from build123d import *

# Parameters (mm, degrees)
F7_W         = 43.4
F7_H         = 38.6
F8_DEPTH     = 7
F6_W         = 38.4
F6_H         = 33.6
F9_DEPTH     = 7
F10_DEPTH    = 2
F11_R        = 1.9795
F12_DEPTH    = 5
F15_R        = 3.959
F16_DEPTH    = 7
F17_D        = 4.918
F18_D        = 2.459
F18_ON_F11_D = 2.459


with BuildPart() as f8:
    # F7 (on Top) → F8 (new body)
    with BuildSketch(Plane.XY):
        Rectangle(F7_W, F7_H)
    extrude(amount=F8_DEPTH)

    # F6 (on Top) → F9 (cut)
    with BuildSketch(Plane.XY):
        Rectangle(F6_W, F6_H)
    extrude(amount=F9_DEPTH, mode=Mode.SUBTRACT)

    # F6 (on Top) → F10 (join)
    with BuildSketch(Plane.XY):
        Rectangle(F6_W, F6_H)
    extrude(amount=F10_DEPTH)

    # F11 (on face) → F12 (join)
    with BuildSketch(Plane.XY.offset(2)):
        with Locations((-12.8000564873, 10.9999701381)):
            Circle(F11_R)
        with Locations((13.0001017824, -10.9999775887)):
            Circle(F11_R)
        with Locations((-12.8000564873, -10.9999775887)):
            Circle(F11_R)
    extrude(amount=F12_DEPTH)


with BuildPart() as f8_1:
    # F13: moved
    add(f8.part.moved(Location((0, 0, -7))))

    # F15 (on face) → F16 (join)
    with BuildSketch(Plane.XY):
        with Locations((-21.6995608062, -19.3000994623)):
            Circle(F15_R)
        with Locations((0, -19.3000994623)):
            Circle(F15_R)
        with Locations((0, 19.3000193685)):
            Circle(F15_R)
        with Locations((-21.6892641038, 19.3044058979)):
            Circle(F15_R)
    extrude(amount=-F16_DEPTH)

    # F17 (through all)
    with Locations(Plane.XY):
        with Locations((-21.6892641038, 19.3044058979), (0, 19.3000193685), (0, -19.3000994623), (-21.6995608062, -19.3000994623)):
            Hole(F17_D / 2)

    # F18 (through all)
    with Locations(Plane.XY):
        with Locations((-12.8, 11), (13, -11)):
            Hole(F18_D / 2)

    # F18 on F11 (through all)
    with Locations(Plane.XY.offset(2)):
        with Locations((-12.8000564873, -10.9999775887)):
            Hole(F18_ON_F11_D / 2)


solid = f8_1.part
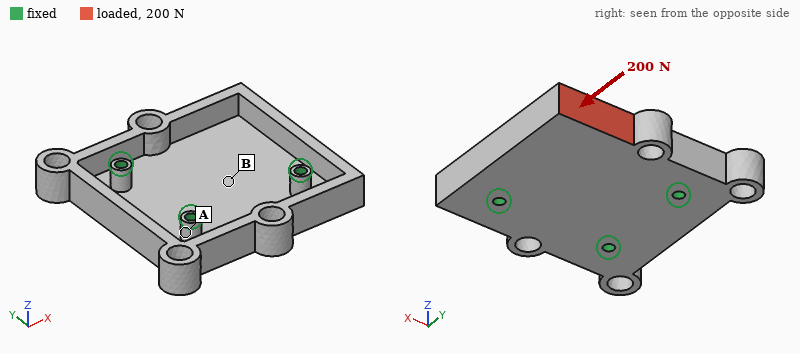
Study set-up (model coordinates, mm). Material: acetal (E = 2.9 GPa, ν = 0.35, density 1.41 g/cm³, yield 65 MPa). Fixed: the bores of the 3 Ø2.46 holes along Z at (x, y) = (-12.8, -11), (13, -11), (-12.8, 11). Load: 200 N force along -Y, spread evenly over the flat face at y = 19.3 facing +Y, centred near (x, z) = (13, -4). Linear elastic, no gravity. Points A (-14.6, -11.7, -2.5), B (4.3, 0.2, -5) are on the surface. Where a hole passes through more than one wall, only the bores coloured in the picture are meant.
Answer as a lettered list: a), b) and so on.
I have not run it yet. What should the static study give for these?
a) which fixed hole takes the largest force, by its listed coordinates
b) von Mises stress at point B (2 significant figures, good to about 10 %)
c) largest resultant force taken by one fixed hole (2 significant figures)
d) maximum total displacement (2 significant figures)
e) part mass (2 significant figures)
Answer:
a) (13, -11)
b) 5.3 MPa
c) 170 N
d) 0.68 mm
e) 8.1 g
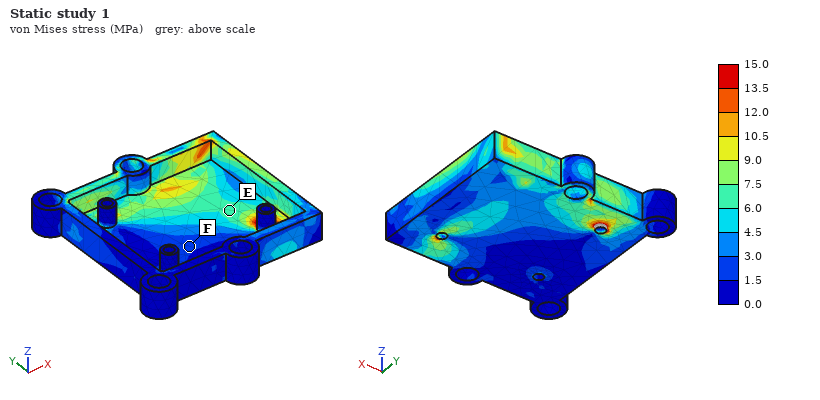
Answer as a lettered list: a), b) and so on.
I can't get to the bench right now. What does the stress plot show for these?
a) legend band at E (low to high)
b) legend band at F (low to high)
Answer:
a) 6.0 to 7.5 MPa
b) 1.5 to 3.0 MPa
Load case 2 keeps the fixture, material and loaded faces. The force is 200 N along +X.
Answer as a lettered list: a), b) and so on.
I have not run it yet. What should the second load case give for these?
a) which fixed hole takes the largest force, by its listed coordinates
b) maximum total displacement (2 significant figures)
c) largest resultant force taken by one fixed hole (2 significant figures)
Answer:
a) (-12.8, 11)
b) 0.72 mm
c) 190 N
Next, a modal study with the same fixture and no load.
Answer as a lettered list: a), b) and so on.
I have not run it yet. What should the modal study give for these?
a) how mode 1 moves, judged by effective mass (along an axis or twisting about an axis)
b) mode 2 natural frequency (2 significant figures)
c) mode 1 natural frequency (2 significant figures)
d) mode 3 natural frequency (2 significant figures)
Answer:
a) along Z
b) 3000 Hz
c) 870 Hz
d) 3000 Hz
